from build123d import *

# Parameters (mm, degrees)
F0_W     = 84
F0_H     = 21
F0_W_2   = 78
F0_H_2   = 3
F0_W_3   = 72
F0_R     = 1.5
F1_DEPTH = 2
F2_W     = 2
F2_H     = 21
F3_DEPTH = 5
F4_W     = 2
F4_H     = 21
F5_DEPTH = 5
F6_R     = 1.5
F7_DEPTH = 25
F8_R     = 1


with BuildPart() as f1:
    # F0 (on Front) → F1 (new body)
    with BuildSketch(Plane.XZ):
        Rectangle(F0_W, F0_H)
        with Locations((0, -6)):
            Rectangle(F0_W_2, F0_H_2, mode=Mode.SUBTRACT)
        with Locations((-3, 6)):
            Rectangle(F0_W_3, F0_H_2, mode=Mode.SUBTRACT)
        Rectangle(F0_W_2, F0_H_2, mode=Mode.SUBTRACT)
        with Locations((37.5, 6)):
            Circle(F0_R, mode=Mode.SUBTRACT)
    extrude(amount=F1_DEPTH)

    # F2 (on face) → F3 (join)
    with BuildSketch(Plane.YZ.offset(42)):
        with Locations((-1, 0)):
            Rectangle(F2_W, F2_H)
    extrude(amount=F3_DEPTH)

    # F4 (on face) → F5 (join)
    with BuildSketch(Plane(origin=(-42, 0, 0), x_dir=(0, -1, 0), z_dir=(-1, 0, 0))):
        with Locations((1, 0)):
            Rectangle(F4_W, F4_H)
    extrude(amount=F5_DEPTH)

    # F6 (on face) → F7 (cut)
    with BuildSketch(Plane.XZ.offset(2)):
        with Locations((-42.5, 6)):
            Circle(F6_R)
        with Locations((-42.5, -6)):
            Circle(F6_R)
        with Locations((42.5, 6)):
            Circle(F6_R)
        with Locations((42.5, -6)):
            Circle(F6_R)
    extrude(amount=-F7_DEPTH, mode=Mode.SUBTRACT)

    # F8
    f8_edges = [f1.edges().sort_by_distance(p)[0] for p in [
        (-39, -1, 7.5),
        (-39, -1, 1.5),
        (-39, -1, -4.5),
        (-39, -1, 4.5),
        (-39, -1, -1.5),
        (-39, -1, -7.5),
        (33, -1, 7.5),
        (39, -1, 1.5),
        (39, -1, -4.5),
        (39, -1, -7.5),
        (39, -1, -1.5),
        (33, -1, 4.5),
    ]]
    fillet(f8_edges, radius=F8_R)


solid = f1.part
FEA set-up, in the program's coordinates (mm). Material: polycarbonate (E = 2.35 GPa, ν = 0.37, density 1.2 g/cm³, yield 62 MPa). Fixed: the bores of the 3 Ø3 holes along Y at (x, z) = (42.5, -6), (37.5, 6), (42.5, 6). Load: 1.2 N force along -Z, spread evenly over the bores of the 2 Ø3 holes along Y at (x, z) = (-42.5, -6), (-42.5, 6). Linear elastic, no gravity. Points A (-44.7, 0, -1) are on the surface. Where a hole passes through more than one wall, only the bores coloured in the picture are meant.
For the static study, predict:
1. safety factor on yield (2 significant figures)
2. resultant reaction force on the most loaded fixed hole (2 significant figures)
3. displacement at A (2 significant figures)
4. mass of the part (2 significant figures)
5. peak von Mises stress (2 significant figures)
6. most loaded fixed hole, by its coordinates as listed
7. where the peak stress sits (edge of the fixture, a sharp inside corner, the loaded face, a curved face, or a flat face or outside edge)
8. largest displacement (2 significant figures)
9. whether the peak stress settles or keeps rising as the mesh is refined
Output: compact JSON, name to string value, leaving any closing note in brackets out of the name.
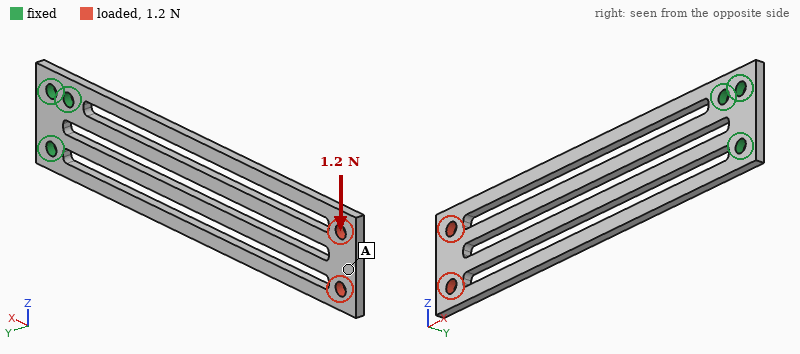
{"safety factor on yield": "9.9", "resultant reaction force on the most loaded fixed hole": "5.3 N", "displacement at A": "1.2 mm", "mass of the part": "3.0 g", "peak von Mises stress": "6.3 MPa", "most loaded fixed hole, by its coordinates as listed": "(42.5, -6)", "where the peak stress sits": "a curved face", "largest displacement": "1.2 mm", "whether the peak stress settles or keeps rising as the mesh is refined": "settles"}
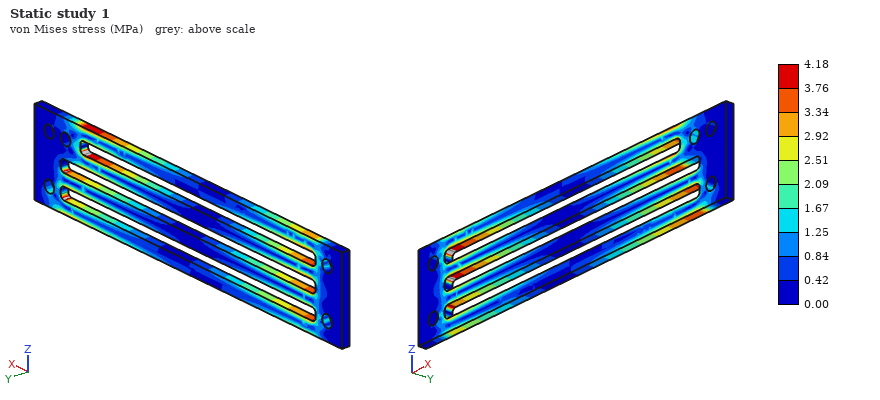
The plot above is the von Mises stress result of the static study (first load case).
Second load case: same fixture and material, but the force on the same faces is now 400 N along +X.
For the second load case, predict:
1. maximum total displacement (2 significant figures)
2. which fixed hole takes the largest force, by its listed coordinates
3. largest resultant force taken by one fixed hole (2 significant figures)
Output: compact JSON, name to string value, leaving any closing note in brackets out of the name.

{"maximum total displacement": "0.66 mm", "which fixed hole takes the largest force, by its listed coordinates": "(42.5, -6)", "largest resultant force taken by one fixed hole": "190 N"}
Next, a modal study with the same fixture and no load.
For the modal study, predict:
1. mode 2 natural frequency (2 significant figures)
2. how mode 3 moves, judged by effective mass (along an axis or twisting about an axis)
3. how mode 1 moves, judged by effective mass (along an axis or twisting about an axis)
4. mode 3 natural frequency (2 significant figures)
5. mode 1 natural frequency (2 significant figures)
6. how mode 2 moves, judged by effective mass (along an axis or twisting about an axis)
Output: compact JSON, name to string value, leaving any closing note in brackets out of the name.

{"mode 2 natural frequency": "150 Hz", "how mode 3 moves, judged by effective mass": "twisting about X", "how mode 1 moves, judged by effective mass": "along Y", "mode 3 natural frequency": "300 Hz", "mode 1 natural frequency": "57 Hz", "how mode 2 moves, judged by effective mass": "along Z"}
